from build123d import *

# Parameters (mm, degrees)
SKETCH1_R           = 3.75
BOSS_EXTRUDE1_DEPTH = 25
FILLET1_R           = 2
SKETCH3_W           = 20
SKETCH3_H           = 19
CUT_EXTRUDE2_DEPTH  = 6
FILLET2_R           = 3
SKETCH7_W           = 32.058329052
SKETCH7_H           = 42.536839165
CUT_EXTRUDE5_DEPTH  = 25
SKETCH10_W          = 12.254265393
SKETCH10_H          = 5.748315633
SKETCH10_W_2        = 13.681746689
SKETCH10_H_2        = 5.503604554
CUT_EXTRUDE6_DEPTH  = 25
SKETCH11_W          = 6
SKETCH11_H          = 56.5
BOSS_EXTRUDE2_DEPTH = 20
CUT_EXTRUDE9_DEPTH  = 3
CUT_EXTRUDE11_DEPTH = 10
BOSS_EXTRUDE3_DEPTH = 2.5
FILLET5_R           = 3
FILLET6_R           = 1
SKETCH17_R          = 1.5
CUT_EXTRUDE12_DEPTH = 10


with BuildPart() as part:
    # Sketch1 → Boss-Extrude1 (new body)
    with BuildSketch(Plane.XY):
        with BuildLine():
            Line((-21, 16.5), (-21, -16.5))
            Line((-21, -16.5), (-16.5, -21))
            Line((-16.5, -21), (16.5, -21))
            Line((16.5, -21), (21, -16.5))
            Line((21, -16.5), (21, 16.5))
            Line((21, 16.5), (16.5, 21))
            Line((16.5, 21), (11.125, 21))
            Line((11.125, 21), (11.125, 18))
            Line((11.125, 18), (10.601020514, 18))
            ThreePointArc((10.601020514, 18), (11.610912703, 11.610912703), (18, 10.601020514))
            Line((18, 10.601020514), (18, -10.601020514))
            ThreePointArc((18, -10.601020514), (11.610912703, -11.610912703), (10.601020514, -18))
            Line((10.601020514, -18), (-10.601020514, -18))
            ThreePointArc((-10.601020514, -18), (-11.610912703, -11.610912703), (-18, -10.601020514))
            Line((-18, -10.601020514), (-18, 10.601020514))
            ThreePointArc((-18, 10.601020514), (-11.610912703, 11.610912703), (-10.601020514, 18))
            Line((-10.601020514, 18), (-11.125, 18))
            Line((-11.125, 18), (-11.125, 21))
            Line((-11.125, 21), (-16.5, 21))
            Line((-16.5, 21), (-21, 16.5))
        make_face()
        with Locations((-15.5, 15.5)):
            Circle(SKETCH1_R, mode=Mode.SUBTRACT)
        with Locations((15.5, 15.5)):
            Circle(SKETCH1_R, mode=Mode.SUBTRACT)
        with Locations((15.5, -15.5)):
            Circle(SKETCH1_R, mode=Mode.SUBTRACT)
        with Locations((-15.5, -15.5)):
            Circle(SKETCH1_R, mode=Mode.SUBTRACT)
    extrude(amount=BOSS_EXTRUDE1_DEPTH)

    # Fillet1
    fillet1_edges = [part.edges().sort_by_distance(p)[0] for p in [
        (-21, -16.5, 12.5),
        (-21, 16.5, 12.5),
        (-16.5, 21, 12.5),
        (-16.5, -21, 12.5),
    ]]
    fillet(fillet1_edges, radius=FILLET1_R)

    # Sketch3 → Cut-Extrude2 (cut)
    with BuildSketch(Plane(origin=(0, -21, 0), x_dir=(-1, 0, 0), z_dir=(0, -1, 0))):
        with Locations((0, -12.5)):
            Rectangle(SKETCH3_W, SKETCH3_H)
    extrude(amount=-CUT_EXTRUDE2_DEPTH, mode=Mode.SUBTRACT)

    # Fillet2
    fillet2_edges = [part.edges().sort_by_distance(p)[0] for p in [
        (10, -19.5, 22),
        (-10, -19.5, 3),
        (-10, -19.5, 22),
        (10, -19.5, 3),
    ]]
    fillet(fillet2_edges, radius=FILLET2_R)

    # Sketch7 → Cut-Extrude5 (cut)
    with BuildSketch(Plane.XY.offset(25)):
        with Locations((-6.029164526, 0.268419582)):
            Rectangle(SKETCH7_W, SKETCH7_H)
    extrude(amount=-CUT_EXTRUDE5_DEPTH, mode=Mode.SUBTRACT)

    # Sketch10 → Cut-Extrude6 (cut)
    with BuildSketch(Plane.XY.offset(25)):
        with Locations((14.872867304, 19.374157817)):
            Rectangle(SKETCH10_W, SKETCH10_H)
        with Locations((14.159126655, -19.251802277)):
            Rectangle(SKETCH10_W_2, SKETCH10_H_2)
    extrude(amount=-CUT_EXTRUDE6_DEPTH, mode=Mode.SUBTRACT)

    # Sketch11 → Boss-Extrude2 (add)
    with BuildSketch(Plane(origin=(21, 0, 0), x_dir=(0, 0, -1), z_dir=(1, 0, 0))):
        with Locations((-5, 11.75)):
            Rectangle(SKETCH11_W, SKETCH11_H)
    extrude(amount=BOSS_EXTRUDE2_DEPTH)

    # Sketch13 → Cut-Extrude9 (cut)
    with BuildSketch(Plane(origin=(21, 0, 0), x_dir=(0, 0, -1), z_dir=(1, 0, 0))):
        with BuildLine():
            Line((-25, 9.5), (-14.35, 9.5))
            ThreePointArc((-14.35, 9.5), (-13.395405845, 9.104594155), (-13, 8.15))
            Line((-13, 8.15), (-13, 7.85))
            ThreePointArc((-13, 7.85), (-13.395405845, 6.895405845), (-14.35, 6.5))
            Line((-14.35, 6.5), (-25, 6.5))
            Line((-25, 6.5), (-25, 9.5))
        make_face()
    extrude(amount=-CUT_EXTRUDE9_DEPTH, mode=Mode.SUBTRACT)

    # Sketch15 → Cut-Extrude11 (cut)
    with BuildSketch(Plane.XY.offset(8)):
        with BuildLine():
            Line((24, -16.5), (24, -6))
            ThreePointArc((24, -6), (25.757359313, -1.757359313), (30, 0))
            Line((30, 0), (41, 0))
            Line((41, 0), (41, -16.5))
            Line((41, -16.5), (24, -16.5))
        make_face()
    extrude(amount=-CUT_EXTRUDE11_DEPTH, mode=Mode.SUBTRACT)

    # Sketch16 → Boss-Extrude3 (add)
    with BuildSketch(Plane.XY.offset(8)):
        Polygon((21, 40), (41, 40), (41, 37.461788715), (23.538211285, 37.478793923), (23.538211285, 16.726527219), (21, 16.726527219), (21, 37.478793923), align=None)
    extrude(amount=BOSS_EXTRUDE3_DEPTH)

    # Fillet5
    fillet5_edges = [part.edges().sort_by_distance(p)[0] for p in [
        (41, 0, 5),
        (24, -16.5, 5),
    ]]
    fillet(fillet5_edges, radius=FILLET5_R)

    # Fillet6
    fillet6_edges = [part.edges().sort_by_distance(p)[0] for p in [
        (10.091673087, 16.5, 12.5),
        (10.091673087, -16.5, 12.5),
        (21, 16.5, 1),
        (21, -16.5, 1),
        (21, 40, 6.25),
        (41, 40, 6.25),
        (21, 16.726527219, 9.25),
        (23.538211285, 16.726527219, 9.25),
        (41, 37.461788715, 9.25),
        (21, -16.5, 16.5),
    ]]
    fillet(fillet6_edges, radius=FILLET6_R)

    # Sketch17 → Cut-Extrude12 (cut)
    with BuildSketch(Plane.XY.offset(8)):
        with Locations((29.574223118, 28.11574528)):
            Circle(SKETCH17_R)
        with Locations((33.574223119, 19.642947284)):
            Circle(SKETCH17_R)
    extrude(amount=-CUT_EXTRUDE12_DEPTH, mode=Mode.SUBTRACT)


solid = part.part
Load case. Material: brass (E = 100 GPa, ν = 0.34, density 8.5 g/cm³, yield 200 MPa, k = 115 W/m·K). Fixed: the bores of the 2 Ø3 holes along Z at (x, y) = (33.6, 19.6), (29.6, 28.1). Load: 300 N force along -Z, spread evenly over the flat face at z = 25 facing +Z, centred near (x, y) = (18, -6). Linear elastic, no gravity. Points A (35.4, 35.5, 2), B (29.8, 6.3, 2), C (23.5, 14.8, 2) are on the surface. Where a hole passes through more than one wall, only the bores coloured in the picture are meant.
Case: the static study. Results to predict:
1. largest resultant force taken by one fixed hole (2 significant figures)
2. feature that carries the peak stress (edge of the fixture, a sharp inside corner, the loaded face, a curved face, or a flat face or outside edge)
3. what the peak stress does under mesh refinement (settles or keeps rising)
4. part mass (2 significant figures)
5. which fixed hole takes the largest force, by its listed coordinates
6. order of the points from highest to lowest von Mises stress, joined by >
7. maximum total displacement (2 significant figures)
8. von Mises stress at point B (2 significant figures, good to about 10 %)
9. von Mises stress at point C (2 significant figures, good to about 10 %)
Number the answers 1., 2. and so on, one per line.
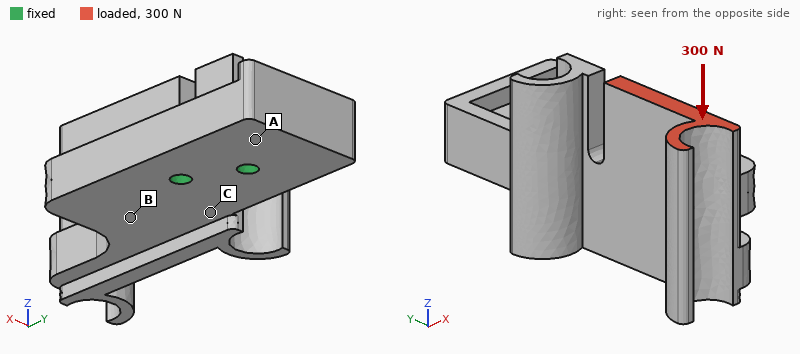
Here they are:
1. 490 N
2. a sharp inside corner
3. keeps rising
4. 72 g
5. (33.6, 19.6)
6. C > B > A
7. 0.15 mm
8. 35 MPa
9. 57 MPa
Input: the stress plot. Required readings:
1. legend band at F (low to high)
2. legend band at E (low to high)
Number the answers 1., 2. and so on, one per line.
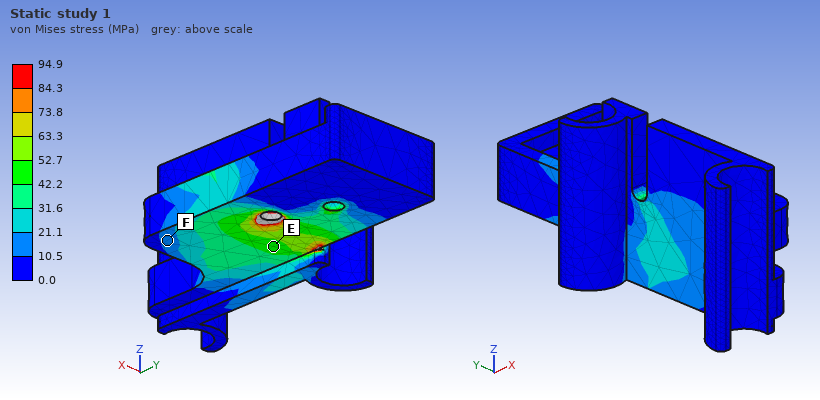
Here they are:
1. 10.5 to 21.1 MPa
2. 42.2 to 52.7 MPa
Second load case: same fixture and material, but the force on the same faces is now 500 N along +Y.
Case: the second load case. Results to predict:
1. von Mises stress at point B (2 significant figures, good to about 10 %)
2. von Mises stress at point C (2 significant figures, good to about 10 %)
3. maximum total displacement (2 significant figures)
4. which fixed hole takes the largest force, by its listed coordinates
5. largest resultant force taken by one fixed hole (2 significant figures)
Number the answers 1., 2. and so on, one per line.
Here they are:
1. 52 MPa
2. 85 MPa
3. 0.22 mm
4. (29.6, 28.1)
5. 860 N
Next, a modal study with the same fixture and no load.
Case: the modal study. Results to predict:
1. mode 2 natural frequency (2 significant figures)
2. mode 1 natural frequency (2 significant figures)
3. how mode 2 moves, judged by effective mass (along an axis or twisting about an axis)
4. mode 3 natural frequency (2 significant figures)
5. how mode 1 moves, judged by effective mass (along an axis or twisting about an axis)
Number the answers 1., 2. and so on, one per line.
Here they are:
1. 2900 Hz
2. 1800 Hz
3. along X
4. 4700 Hz
5. along Z
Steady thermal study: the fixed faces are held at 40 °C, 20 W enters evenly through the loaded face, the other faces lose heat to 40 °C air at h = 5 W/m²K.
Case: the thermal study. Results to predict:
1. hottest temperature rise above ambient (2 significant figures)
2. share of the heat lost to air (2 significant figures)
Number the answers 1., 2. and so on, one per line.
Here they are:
1. 84 K
2. 3.8 %
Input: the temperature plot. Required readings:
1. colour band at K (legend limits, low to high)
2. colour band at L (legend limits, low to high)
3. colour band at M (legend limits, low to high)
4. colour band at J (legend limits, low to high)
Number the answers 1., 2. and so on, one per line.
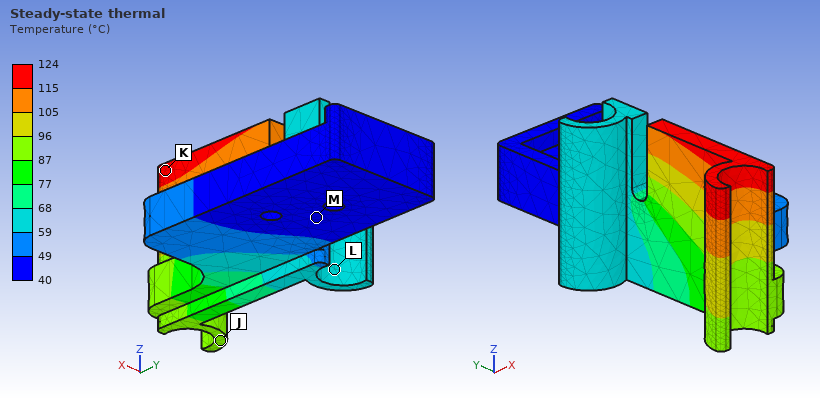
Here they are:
1. 115 to 124 °C
2. 59 to 68 °C
3. 40 to 49 °C
4. 87 to 96 °C
